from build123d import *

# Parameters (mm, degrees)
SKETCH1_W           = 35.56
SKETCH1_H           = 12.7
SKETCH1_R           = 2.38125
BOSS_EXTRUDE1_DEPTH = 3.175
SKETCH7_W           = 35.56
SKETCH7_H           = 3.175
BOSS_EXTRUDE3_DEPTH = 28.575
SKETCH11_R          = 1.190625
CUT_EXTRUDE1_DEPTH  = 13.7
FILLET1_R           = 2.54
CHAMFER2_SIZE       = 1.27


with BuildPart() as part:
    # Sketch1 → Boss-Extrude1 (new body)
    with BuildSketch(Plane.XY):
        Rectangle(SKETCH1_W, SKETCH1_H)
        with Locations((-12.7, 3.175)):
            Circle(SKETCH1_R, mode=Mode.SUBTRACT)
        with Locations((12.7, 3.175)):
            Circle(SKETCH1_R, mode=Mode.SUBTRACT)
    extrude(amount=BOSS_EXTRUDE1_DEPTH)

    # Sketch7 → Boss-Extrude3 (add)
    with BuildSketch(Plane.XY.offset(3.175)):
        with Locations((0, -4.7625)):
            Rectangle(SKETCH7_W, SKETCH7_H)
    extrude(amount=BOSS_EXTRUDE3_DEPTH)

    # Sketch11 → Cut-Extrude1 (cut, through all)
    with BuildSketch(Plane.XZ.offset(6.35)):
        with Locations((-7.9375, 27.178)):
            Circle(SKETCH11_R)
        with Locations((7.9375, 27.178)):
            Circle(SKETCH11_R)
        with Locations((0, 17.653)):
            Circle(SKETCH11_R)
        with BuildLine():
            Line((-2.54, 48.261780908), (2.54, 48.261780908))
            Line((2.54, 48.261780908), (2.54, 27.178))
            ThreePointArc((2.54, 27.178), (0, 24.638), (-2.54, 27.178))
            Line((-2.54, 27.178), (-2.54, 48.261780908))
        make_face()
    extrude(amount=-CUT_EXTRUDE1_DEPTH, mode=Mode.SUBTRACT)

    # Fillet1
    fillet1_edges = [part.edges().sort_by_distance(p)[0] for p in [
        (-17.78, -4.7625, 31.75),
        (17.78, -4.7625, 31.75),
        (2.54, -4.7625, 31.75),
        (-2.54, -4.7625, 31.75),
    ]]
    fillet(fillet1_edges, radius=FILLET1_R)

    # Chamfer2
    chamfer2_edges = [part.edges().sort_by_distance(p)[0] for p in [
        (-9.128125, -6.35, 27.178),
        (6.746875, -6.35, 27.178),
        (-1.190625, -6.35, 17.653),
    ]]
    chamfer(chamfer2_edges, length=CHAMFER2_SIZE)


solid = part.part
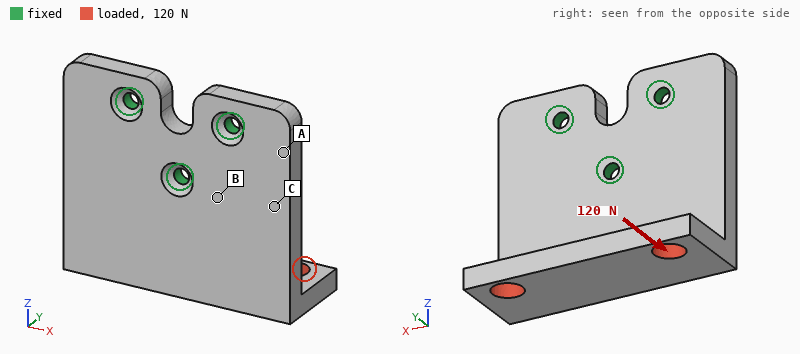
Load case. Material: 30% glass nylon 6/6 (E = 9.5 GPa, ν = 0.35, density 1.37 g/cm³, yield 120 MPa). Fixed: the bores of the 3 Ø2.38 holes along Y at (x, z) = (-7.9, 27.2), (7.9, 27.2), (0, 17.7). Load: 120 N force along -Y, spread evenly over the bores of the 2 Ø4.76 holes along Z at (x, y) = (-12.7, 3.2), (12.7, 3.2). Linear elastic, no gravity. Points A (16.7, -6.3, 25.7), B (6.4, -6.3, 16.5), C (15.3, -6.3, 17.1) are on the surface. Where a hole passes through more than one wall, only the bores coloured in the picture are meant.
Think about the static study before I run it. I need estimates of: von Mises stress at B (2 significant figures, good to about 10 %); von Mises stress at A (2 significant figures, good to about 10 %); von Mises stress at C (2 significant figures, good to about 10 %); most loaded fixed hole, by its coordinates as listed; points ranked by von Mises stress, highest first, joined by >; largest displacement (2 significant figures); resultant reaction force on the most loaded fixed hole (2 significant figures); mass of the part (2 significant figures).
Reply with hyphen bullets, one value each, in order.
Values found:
- 27 MPa
- 6.7 MPa
- 17 MPa
- (0, 17.7)
- B > C > A
- 0.46 mm
- 250 N
- 6.0 g
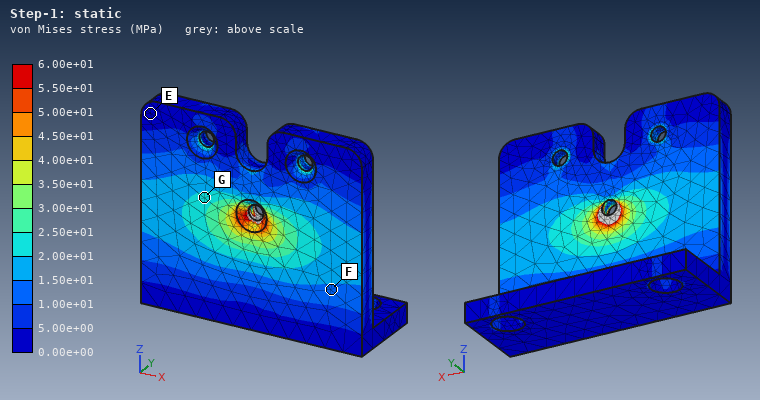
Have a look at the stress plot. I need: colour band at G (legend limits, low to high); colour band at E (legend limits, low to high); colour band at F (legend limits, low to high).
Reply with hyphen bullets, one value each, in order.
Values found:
- 2.00e+01 to 2.50e+01 MPa
- 0.00e+00 to 5.00e+00 MPa
- 1.00e+01 to 1.50e+01 MPa
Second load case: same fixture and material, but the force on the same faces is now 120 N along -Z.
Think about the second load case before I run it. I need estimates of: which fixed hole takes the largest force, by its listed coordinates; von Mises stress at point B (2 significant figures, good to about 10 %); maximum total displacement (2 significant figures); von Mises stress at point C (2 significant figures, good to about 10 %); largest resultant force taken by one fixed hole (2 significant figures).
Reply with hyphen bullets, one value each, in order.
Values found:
- (0, 17.7)
- 13 MPa
- 0.34 mm
- 11 MPa
- 120 N
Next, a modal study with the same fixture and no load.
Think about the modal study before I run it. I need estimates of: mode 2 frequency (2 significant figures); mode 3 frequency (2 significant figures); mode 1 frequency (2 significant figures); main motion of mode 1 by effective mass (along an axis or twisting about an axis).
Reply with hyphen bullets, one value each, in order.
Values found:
- 2300 Hz
- 6100 Hz
- 1800 Hz
- along Y
